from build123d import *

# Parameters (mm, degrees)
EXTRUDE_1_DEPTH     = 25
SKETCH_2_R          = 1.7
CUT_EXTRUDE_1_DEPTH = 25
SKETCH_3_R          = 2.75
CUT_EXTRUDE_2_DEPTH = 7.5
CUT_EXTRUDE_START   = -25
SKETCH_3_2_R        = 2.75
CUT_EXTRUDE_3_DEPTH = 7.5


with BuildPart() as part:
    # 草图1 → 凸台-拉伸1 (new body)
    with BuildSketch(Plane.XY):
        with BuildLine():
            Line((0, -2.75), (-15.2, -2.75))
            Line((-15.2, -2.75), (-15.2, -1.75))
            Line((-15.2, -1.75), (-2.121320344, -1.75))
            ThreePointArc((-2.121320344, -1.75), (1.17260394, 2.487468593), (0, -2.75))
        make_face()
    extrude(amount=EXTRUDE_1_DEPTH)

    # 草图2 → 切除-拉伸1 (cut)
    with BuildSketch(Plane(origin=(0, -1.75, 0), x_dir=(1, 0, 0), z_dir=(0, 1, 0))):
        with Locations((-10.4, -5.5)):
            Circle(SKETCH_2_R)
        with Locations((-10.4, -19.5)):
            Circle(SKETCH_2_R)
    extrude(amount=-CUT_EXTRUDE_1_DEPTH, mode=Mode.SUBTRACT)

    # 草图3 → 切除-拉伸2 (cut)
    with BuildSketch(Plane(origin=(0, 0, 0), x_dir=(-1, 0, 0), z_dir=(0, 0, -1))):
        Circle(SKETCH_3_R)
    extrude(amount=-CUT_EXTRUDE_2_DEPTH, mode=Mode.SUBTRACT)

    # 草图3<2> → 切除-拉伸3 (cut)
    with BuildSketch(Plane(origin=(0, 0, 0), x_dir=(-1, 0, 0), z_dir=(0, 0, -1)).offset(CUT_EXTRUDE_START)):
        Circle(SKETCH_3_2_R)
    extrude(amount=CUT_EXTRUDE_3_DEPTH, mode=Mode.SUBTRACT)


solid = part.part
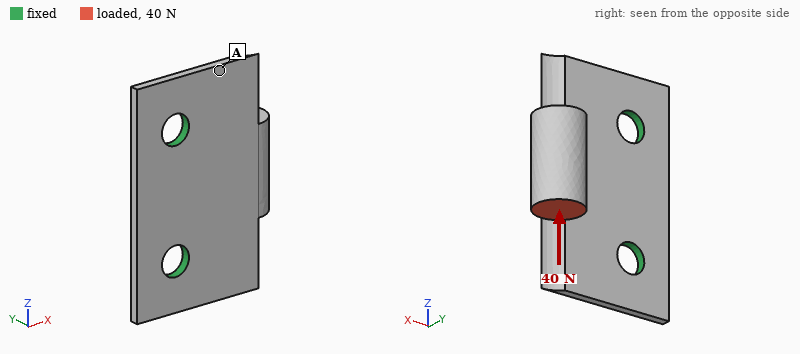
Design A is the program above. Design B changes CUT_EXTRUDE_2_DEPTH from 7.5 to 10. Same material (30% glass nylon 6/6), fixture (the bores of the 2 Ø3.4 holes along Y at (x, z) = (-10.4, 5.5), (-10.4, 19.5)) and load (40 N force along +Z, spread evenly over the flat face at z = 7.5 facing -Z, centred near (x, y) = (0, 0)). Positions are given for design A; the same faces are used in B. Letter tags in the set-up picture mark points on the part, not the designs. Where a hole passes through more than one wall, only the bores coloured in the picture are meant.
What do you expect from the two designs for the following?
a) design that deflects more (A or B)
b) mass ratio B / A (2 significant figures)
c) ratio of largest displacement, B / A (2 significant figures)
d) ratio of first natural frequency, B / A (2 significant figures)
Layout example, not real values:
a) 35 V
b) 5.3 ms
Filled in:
a) B
b) 0.89
c) 1.4
d) 1.1
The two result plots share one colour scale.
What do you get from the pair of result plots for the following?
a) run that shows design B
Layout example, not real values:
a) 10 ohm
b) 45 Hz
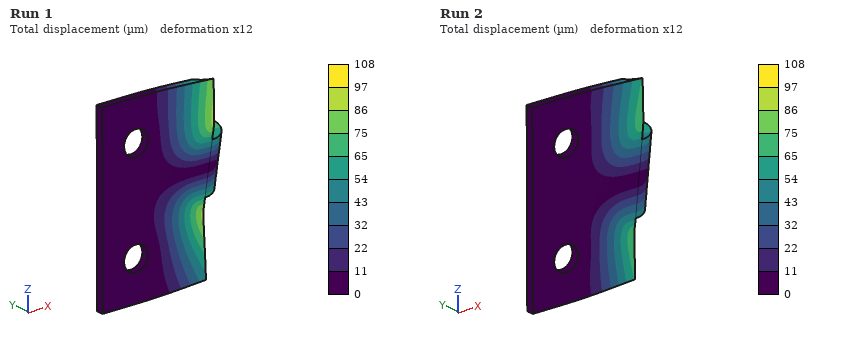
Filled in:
a) Run 1
